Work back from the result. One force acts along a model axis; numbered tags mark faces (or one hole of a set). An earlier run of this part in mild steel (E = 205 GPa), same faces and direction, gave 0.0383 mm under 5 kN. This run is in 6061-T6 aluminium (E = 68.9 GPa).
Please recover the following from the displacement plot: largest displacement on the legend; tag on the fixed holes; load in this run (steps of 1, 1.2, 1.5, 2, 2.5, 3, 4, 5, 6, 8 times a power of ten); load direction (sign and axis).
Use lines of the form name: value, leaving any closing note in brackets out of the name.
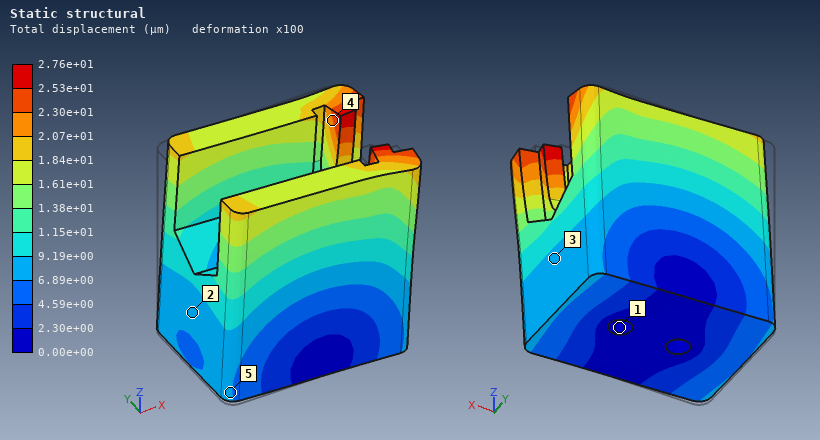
largest displacement on the legend: 2.76e+01 µm
tag on the fixed holes: 1
load in this run: 1.2 kN
load direction: +X
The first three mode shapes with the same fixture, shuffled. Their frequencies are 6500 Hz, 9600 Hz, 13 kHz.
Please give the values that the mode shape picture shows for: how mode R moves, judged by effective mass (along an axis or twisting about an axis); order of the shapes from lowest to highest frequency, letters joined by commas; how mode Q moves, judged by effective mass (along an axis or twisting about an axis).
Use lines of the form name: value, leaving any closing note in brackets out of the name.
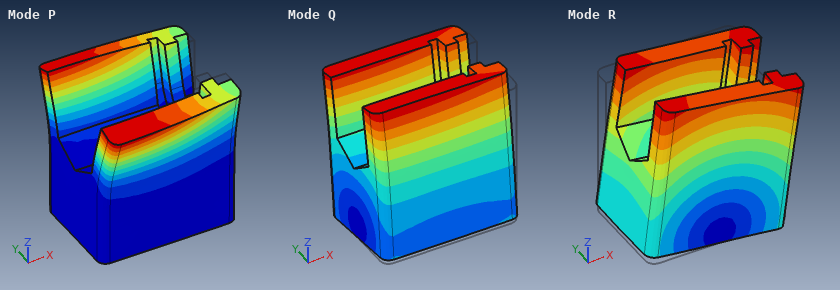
how mode R moves, judged by effective mass: along X
order of the shapes from lowest to highest frequency, letters joined by commas: Q, R, P
how mode Q moves, judged by effective mass: along Y
